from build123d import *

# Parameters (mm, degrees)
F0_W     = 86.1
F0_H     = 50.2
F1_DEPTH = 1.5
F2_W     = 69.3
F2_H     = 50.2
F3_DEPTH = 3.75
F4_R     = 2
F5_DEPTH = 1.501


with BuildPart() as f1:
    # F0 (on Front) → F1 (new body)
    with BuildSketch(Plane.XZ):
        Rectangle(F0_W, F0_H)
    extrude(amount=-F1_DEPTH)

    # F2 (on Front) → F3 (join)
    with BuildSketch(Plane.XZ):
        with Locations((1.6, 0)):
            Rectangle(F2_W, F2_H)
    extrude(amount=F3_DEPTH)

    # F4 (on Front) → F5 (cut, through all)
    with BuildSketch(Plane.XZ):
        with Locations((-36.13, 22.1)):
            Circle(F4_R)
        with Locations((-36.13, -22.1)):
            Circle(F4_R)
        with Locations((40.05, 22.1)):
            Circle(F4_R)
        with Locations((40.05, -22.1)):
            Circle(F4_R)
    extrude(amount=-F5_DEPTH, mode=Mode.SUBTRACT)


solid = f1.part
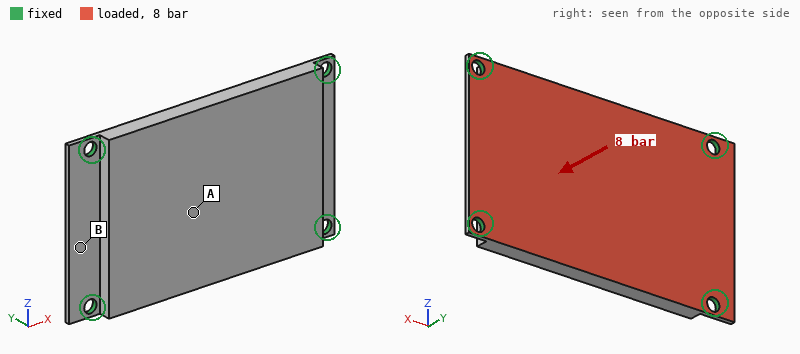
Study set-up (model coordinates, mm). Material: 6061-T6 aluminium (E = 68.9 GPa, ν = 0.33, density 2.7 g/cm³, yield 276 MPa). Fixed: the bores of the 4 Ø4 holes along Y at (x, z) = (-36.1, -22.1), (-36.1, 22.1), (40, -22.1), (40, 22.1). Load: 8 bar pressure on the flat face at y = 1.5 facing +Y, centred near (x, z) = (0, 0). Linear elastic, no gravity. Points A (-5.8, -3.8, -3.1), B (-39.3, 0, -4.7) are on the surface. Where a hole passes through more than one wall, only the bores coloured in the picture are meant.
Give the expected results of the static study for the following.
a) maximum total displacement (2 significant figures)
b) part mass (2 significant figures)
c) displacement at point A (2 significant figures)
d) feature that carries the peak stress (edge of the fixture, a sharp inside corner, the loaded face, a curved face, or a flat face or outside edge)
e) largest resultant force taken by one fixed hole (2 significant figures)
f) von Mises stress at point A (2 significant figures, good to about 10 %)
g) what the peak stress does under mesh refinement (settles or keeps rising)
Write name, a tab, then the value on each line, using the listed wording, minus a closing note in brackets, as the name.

maximum total displacement	0.23 mm
part mass	53 g
displacement at point A	0.21 mm
feature that carries the peak stress	edge of the fixture
largest resultant force taken by one fixed hole	2.0 kN
von Mises stress at point A	68 MPa
what the peak stress does under mesh refinement	keeps rising
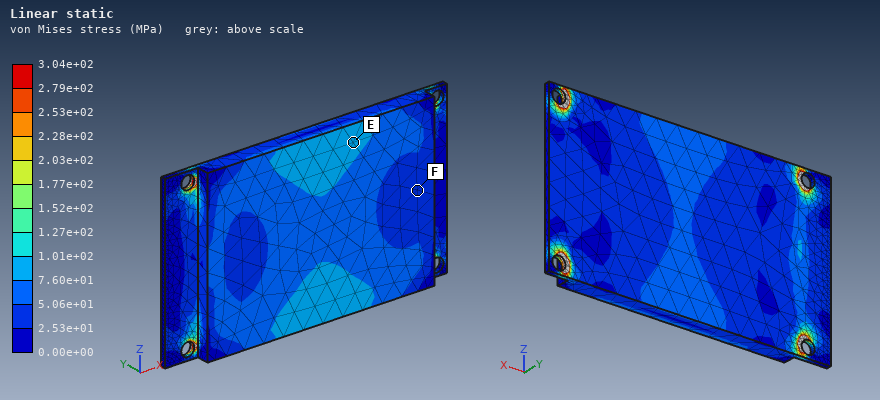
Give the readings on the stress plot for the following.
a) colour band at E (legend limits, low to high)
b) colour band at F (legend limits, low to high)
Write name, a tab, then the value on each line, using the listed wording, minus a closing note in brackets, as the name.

colour band at E	7.60e+01 to 1.01e+02 MPa
colour band at F	2.53e+01 to 5.06e+01 MPa
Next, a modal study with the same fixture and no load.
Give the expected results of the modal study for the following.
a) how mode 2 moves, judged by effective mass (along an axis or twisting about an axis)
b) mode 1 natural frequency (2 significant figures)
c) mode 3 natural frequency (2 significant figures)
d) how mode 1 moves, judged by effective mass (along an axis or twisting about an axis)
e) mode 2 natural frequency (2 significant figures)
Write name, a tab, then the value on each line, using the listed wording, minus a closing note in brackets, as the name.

how mode 2 moves, judged by effective mass	twisting about X
mode 1 natural frequency	2800 Hz
mode 3 natural frequency	6800 Hz
how mode 1 moves, judged by effective mass	along Y
mode 2 natural frequency	5000 Hz
